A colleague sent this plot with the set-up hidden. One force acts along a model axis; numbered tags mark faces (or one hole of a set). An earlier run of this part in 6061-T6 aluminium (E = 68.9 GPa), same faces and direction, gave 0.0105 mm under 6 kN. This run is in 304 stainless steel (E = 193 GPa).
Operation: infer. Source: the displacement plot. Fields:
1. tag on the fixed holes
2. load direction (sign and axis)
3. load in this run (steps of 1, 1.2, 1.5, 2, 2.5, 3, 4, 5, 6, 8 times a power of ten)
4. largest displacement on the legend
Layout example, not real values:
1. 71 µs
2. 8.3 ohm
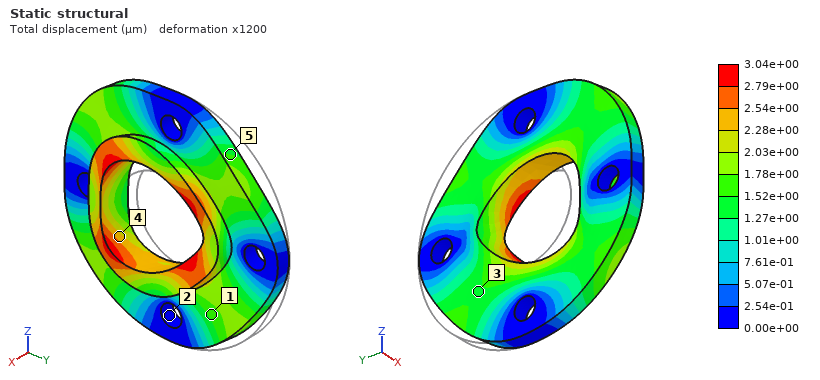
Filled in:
1. 2
2. -Y
3. 5 kN
4. 3.04e+00 µm
